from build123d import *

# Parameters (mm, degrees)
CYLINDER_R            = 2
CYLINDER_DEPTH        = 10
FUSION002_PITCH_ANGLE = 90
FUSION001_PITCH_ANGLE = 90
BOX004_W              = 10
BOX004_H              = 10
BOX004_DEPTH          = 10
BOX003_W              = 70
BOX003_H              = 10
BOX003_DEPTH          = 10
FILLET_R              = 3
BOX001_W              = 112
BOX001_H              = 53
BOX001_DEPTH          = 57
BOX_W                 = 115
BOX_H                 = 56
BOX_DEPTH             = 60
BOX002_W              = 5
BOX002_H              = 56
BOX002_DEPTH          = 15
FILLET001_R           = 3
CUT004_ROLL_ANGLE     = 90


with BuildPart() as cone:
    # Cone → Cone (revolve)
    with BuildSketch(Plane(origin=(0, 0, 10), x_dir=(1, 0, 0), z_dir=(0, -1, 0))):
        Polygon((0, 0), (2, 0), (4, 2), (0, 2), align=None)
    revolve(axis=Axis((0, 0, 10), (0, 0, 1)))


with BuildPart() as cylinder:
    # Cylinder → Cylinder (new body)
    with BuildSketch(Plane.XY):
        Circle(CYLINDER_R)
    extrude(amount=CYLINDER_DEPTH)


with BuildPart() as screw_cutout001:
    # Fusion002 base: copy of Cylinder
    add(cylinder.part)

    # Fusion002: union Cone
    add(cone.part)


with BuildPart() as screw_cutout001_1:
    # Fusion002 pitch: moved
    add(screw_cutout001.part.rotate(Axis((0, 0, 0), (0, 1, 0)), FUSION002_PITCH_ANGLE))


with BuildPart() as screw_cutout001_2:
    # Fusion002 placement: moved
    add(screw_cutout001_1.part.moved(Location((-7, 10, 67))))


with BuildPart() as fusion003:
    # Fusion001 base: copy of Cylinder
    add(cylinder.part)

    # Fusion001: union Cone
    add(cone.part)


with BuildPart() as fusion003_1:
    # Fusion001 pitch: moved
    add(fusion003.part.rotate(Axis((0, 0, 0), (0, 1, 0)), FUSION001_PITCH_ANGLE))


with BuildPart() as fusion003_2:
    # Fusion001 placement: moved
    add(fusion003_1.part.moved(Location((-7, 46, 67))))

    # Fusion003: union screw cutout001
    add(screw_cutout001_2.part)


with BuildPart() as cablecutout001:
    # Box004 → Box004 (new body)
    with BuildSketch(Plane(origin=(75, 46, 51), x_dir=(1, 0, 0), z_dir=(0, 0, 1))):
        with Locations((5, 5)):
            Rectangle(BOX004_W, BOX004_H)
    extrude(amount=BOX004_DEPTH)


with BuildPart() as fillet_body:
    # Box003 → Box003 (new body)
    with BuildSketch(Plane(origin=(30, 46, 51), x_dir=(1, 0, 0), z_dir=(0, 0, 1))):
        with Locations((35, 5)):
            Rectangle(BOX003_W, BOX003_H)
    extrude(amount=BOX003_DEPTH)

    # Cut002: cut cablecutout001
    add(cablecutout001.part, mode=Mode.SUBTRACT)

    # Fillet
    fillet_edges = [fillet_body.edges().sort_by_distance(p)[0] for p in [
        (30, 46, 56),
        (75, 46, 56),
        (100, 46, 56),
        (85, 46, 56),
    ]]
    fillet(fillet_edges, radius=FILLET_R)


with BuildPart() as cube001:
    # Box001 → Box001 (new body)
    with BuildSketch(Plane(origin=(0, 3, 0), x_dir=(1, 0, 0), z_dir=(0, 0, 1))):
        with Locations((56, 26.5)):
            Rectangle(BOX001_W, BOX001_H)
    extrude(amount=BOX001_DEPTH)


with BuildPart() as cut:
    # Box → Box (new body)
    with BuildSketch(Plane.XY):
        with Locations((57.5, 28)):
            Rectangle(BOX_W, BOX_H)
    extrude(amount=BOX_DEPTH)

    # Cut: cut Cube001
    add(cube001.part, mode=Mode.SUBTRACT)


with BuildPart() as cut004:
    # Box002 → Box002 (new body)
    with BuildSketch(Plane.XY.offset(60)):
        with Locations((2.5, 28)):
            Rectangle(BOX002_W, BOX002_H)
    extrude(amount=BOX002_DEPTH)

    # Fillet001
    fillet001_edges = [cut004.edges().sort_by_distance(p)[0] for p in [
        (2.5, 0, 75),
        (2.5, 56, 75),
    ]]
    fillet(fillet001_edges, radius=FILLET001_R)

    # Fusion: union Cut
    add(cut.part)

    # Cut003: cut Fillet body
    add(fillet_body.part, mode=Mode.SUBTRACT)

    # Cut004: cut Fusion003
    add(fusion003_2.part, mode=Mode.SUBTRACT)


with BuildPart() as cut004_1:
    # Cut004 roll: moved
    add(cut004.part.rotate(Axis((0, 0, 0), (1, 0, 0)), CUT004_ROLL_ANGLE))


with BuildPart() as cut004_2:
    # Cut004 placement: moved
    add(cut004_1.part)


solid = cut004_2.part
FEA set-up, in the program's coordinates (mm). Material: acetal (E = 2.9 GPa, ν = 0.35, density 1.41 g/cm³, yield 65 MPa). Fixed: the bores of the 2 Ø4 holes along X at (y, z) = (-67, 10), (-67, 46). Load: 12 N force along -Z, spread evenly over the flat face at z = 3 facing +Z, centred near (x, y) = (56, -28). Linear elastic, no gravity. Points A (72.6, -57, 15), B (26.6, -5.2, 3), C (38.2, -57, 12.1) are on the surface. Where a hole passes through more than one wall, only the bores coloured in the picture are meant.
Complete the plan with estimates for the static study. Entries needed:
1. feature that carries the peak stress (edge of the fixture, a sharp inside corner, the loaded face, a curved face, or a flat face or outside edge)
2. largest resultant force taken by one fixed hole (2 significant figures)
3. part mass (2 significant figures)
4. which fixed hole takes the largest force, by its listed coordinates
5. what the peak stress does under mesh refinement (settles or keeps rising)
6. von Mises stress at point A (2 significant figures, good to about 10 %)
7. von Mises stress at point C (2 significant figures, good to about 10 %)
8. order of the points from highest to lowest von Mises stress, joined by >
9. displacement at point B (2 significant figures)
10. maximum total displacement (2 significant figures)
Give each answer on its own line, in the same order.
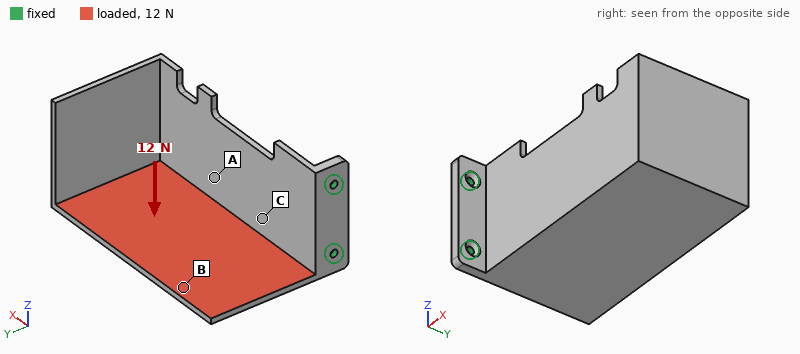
a sharp inside corner
24 N
71 g
(-67, 46)
keeps rising
1.3 MPa
2.1 MPa
C > A > B
1.0 mm
1.5 mm
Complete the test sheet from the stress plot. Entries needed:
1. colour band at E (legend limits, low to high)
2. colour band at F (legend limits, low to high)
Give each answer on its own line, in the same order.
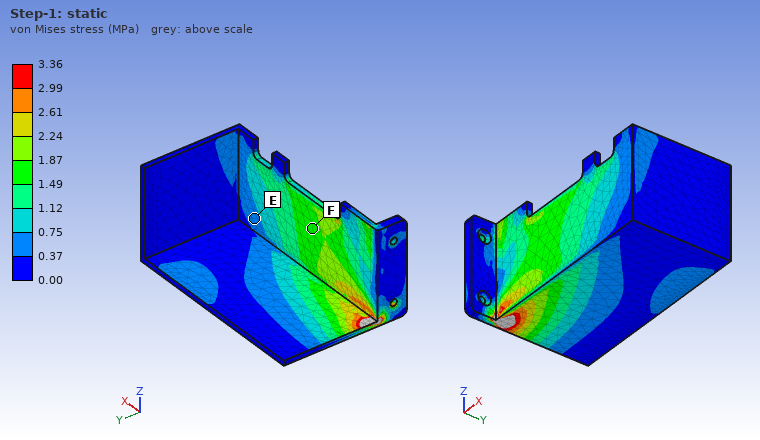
0.37 to 0.75 MPa
1.49 to 1.87 MPa
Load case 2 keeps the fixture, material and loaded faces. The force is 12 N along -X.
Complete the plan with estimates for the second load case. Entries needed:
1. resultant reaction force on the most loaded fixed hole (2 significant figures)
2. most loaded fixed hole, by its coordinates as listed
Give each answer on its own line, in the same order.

14 N
(-67, 10)
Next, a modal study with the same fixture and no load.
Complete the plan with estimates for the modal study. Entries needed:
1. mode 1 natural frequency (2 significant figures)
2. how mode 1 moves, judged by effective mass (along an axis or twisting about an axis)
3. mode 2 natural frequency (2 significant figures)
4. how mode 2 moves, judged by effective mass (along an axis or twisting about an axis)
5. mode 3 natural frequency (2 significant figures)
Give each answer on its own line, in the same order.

46 Hz
along Y
78 Hz
along Z
230 Hz
